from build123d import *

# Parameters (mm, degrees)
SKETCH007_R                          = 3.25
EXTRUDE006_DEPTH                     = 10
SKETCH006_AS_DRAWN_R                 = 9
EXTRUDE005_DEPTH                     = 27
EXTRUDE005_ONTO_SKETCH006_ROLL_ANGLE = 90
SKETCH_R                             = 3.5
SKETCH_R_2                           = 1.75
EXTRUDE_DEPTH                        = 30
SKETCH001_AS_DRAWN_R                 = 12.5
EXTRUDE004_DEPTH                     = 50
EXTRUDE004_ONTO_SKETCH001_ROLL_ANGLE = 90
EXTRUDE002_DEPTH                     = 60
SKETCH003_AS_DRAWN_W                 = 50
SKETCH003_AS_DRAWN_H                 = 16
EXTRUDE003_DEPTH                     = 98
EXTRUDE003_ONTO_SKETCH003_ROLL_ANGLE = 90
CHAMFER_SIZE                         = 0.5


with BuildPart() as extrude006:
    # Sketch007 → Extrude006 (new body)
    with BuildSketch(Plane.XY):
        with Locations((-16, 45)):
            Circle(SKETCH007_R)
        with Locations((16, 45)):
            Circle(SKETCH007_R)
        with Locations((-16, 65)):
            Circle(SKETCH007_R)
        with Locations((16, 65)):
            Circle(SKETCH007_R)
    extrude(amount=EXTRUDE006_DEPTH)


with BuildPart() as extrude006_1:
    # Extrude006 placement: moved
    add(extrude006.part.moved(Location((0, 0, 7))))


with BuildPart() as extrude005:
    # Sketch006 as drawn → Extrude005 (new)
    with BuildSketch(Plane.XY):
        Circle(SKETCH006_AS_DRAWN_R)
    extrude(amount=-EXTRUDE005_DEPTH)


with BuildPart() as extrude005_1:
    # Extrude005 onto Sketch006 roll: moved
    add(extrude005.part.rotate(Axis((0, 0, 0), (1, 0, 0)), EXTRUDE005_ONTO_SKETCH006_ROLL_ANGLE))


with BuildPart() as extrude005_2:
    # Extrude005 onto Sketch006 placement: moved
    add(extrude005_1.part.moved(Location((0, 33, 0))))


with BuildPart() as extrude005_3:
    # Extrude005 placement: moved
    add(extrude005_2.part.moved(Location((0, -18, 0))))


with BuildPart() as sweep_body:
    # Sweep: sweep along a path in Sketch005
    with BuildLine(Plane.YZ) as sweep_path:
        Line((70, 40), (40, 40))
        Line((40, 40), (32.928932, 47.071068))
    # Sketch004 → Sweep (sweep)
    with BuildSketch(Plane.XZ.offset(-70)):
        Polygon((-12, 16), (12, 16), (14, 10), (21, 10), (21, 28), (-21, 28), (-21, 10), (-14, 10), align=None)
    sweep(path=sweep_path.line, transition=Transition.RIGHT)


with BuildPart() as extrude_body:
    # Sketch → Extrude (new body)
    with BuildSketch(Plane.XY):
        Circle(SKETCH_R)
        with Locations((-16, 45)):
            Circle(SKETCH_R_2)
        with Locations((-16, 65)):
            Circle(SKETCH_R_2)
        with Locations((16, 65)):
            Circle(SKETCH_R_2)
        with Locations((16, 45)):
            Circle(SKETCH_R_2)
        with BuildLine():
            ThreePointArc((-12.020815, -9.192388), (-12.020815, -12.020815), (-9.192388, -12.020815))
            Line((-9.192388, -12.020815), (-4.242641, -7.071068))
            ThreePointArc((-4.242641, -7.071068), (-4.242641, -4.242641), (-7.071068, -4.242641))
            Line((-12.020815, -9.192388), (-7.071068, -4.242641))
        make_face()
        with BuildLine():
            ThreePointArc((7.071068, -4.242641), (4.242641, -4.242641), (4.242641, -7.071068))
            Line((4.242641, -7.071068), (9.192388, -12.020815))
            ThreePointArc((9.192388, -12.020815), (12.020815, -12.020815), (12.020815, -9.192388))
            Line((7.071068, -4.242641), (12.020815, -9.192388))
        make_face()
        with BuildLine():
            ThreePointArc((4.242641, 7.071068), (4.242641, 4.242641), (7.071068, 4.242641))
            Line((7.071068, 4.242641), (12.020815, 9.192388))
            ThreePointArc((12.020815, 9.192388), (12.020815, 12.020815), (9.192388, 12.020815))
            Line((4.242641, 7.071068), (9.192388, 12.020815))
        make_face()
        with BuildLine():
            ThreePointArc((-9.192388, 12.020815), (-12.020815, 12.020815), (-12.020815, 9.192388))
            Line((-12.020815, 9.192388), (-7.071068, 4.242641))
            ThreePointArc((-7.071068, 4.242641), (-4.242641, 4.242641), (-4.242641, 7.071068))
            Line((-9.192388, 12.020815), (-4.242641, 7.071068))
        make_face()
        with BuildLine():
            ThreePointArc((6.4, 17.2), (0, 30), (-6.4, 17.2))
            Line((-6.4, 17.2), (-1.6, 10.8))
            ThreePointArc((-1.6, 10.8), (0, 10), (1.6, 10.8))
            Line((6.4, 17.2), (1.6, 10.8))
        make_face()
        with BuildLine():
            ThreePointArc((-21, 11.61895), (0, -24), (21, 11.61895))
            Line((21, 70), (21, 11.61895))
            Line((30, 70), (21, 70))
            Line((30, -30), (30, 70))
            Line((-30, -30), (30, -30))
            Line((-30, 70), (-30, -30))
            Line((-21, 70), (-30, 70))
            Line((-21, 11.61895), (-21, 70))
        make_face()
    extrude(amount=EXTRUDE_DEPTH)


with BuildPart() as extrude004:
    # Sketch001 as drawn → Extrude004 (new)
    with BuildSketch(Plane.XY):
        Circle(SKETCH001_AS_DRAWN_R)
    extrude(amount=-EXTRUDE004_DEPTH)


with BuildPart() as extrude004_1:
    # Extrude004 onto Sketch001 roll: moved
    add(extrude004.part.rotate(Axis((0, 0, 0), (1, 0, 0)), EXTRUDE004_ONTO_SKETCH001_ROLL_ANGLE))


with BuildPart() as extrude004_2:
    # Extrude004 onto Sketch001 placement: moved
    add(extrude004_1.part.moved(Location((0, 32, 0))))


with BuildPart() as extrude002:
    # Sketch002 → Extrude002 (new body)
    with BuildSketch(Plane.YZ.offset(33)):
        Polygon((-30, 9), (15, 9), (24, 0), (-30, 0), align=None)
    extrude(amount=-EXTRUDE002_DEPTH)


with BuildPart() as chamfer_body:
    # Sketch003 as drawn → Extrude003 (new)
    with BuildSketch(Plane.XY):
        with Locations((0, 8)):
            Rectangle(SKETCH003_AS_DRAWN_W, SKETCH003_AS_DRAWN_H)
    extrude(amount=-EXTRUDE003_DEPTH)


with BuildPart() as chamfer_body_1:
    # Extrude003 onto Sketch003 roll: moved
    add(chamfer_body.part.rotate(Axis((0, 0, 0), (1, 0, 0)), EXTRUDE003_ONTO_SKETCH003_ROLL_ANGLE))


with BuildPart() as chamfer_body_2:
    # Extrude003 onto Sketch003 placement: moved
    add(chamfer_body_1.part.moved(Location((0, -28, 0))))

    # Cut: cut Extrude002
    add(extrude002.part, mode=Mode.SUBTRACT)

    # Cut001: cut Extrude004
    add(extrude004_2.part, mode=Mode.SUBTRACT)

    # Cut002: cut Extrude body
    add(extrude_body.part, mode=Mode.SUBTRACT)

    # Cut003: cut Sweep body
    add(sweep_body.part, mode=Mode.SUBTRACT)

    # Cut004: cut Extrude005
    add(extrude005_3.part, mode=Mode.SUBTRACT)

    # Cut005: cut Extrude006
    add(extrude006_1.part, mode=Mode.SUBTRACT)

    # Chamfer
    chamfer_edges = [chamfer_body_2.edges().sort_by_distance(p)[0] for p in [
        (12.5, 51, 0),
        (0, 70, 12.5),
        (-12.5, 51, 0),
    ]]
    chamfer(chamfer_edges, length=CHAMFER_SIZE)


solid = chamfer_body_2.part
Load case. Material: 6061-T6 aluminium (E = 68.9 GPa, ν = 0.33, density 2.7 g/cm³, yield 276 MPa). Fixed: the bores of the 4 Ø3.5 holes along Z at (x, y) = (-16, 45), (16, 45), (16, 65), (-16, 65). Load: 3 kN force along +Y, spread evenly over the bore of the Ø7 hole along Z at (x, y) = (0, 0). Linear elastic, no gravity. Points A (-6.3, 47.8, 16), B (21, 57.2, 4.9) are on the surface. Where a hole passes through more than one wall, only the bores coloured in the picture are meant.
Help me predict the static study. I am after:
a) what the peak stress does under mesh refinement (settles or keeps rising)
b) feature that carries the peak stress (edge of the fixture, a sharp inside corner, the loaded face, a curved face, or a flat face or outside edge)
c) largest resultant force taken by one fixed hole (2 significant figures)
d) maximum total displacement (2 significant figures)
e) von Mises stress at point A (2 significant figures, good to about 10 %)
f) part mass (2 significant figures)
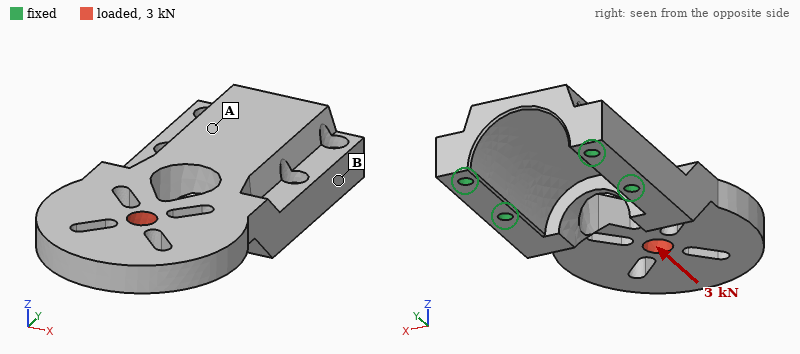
keeps rising
edge of the fixture
1.0 kN
0.11 mm
16 MPa
74 g
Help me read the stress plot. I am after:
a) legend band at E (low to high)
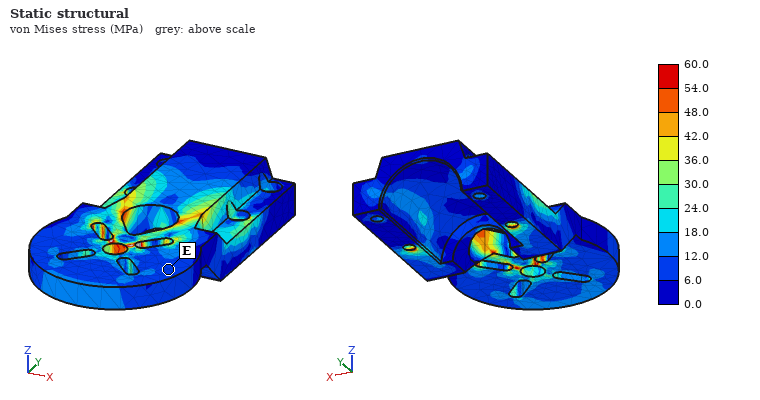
6.0 to 12.0 MPa
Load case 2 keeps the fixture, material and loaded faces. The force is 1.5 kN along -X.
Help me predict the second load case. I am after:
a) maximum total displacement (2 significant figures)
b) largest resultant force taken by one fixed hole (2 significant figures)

81 µm
1.7 kN
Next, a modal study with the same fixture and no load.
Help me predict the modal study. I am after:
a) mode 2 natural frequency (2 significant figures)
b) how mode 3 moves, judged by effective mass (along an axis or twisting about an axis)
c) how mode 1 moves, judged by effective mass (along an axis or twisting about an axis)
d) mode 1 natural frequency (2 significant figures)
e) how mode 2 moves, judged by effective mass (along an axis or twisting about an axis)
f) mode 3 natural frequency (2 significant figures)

3900 Hz
along X
along Z
1900 Hz
along X
5900 Hz
